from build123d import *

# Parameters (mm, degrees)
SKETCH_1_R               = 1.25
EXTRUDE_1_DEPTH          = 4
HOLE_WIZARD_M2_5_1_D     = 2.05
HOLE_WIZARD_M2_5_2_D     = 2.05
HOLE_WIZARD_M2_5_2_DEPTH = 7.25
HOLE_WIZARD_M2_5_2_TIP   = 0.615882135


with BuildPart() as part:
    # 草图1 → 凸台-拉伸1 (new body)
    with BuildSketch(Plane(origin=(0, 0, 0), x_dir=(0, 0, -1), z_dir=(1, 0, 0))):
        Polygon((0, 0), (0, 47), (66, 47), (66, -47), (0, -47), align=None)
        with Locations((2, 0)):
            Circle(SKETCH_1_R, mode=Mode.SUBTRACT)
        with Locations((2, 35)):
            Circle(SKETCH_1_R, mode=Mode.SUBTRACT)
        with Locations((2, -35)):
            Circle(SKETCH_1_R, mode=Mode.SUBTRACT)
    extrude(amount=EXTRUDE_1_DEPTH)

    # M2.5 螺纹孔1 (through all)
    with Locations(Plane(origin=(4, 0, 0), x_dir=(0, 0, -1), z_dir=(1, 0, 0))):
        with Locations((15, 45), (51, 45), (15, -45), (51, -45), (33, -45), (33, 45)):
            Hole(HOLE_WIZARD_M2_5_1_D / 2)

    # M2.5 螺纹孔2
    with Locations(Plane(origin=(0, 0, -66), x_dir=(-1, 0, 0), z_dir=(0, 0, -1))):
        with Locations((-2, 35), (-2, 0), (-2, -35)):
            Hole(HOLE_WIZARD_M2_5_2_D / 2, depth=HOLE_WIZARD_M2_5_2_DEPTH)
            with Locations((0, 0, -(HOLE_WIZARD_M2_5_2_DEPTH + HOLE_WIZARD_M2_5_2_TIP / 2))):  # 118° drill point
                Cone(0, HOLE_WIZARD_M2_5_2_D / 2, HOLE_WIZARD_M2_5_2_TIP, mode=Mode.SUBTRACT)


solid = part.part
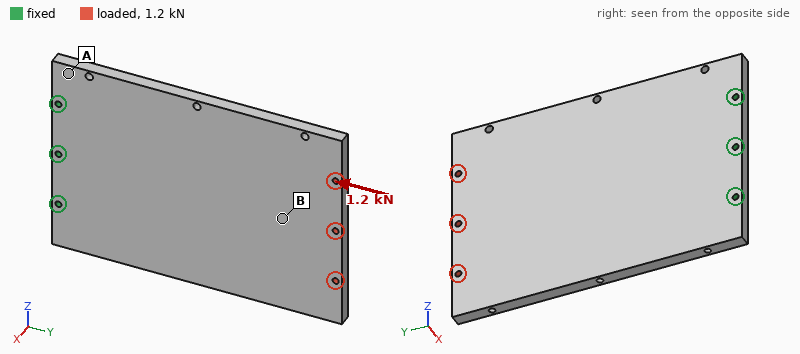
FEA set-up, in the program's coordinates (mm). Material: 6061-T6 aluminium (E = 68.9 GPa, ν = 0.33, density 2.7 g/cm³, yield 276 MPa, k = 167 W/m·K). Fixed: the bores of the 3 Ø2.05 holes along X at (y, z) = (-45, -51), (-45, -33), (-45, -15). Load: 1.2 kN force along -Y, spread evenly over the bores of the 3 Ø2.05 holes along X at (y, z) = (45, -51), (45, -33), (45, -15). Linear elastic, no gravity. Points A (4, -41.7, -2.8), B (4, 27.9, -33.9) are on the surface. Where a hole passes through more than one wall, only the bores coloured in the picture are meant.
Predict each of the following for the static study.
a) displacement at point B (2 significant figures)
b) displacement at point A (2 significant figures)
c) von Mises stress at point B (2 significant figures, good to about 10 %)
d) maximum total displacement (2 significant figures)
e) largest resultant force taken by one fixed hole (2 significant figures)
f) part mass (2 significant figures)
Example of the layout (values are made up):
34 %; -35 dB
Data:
6.4 µm; 2.4 µm; 5.8 MPa; 9.4 µm; 420 N; 66 g
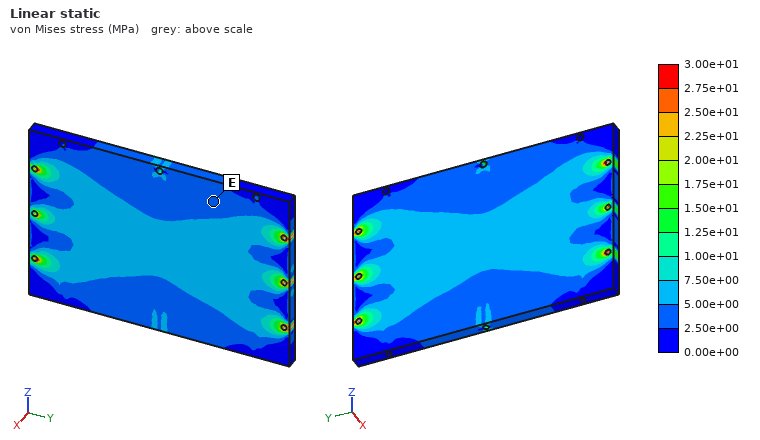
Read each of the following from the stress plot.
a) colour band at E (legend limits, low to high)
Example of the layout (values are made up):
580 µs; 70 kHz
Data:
2.50e+00 to 5.00e+00 MPa
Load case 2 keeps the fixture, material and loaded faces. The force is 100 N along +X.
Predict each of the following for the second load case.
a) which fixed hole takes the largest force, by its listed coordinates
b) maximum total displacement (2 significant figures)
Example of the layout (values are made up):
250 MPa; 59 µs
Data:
(-45, -33); 1.2 mm
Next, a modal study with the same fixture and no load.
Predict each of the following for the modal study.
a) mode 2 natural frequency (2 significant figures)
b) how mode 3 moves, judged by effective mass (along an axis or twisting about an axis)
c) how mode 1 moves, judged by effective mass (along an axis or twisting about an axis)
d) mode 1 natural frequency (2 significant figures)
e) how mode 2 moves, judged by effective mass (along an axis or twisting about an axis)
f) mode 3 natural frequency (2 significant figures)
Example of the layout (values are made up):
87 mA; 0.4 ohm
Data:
1100 Hz; along X; along X; 360 Hz; twisting about Y; 2200 Hz
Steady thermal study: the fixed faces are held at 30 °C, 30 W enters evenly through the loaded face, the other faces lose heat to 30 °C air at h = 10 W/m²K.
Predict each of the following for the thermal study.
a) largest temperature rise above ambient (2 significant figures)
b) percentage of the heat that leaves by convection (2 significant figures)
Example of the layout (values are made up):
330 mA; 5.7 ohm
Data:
66 K; 14 %
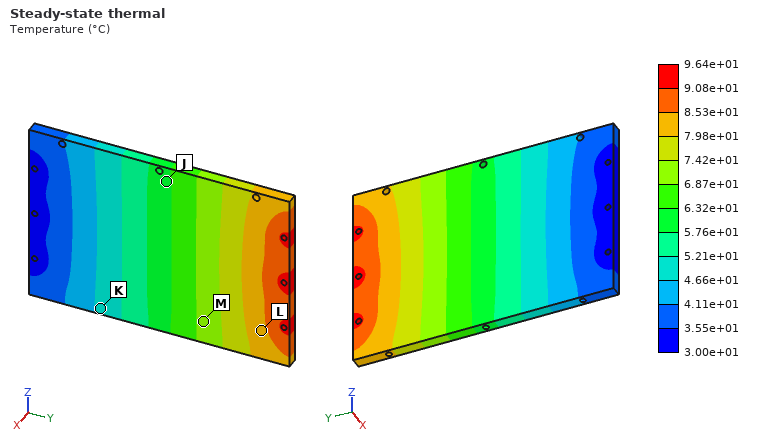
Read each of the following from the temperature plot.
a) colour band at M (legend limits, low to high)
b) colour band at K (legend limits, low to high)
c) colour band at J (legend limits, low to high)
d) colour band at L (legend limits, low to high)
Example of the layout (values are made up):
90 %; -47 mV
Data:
6.87e+01 to 7.42e+01 °C; 4.66e+01 to 5.21e+01 °C; 5.76e+01 to 6.32e+01 °C; 7.98e+01 to 8.53e+01 °C
